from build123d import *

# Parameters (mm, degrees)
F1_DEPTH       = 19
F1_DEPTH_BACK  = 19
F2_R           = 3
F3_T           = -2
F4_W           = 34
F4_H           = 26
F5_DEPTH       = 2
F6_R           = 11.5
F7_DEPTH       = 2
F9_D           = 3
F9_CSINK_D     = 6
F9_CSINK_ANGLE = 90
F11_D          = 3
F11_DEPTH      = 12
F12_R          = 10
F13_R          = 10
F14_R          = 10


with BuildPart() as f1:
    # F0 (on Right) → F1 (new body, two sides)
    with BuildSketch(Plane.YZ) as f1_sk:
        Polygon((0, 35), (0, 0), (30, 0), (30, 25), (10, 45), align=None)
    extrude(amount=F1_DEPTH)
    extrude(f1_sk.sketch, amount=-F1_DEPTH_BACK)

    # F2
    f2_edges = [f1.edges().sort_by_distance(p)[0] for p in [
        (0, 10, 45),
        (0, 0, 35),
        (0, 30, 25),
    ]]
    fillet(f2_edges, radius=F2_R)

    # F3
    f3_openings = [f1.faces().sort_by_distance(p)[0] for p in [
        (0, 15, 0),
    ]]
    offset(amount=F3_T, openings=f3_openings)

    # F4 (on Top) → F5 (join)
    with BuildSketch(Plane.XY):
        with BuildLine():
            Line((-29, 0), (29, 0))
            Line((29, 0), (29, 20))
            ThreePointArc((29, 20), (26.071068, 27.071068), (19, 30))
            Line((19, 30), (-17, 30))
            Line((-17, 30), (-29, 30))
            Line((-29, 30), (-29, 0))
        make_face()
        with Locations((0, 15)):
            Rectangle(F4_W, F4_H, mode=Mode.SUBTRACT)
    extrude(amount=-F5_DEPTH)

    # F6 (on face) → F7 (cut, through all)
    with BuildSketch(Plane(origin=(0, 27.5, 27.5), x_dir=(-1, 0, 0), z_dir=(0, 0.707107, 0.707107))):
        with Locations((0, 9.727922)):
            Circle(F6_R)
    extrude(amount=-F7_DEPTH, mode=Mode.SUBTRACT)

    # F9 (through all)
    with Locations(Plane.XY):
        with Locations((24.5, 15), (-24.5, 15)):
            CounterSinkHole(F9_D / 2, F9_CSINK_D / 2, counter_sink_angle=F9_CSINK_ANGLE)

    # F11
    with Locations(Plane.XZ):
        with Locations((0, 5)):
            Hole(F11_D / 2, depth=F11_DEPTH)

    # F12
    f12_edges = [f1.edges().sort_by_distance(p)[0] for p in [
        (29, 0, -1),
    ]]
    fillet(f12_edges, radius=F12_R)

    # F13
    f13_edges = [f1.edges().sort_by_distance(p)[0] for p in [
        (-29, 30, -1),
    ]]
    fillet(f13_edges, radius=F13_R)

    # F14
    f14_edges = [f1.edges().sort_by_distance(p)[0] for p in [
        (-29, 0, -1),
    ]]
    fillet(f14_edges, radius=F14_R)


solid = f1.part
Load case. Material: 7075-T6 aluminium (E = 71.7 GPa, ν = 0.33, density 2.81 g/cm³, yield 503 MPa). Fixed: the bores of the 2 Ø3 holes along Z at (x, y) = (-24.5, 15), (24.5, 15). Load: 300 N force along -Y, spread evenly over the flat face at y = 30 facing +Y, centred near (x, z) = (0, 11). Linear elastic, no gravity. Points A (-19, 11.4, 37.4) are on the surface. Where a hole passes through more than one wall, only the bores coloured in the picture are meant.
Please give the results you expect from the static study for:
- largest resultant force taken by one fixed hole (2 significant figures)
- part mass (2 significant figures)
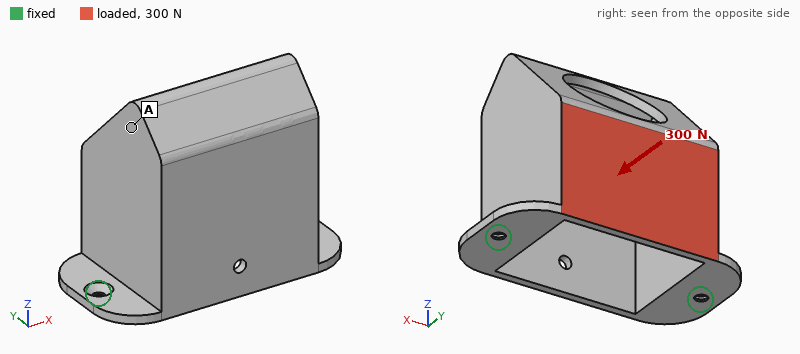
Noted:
150 N
33 g
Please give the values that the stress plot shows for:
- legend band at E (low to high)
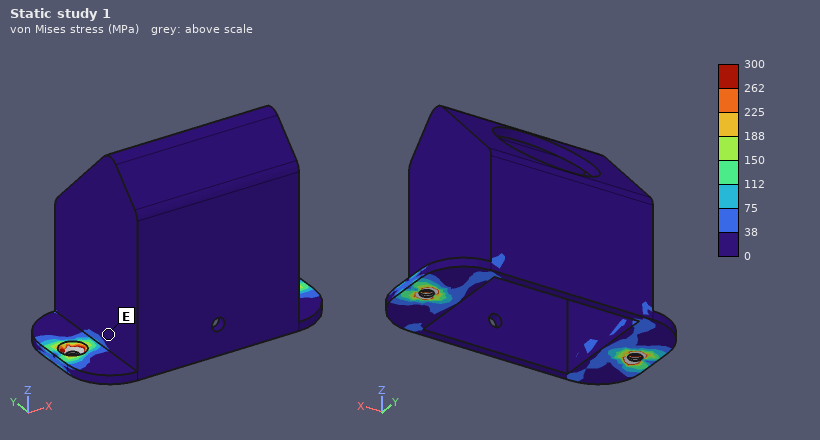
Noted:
0 to 38 MPa
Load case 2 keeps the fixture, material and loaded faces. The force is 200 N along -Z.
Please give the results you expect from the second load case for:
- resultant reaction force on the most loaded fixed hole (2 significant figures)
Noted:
120 N
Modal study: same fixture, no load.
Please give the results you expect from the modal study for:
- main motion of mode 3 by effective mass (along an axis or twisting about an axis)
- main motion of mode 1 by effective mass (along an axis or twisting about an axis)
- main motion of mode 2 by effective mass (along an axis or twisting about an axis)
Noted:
along Z
along Y
along X
